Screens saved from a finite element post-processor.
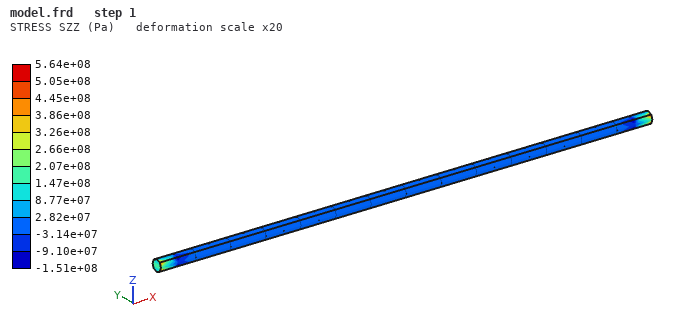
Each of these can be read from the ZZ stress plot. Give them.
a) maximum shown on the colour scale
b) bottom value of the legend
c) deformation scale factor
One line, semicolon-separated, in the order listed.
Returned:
5.64e+08 Pa; -1.51e+08 Pa; 20
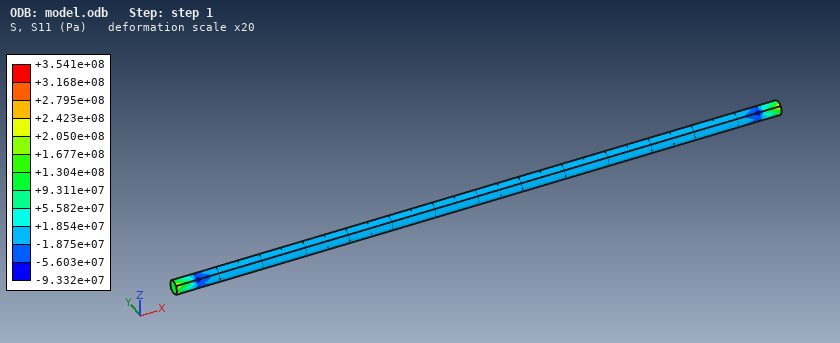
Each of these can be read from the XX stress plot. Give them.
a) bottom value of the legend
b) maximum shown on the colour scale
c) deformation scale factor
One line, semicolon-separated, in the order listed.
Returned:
-9.332e+07 Pa; +3.541e+08 Pa; 20
